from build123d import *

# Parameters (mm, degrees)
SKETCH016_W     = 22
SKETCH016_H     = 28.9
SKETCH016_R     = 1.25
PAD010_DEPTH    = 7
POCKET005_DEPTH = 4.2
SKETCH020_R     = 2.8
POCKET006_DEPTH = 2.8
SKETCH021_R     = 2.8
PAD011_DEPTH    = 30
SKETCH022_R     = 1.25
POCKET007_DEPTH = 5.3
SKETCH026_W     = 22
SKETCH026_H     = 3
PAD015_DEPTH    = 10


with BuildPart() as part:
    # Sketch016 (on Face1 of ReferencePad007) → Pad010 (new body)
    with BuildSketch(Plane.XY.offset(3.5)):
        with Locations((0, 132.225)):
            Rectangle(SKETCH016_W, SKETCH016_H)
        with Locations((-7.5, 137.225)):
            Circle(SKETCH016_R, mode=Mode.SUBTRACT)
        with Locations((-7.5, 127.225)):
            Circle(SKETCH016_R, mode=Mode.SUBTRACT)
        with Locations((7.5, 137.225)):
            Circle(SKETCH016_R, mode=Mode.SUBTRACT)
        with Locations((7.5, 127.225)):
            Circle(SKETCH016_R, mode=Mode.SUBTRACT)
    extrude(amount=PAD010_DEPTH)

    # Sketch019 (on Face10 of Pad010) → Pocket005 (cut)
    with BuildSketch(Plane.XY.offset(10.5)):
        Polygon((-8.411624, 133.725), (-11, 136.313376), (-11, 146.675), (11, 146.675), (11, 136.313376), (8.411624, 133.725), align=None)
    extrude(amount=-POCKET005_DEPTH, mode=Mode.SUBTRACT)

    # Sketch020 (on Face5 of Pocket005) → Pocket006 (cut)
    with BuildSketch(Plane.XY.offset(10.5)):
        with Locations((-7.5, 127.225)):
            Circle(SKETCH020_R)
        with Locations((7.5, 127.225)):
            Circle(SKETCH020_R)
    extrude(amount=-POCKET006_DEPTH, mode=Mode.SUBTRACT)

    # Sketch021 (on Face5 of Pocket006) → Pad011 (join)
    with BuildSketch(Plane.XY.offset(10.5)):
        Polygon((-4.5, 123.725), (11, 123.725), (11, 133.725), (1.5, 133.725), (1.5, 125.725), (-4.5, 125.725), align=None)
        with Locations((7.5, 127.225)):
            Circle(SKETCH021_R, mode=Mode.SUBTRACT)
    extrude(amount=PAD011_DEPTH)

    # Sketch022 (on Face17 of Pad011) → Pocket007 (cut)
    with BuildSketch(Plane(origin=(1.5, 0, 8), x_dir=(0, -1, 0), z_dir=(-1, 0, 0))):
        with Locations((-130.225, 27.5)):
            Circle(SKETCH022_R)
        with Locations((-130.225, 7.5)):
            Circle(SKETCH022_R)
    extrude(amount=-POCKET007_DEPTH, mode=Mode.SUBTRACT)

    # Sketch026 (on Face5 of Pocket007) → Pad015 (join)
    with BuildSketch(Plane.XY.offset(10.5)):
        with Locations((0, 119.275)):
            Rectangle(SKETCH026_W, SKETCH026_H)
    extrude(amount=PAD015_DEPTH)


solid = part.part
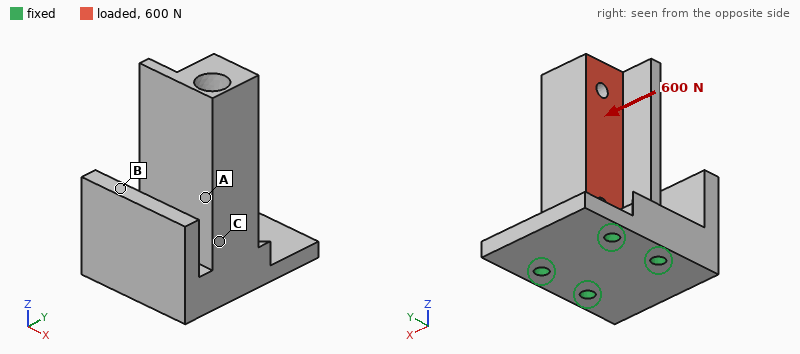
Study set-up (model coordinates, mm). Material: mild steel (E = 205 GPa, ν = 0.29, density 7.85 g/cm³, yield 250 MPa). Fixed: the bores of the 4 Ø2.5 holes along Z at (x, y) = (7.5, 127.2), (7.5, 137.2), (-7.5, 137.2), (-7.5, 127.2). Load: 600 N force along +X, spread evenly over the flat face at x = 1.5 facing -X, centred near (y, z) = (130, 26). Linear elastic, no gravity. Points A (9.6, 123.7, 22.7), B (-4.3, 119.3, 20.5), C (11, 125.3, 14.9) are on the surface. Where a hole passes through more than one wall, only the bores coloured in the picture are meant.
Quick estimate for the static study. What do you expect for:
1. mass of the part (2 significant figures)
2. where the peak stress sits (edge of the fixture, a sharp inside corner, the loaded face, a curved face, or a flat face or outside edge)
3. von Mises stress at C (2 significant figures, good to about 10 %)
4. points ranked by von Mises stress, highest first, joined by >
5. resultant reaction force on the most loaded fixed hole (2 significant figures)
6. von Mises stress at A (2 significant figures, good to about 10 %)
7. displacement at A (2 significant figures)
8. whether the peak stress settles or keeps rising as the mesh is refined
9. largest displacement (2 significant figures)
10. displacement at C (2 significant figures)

48 g
edge of the fixture
48 MPa
C > A > B
720 N
25 MPa
8.6 µm
keeps rising
23 µm
4.5 µm
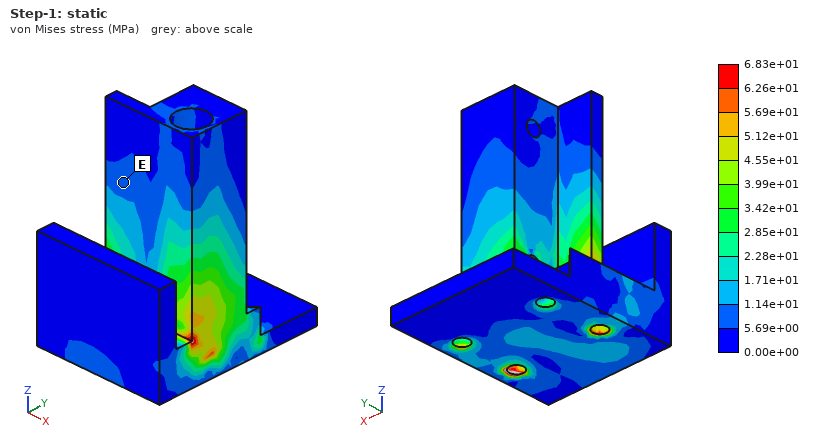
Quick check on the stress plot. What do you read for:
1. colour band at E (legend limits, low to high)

5.69e+00 to 1.14e+01 MPa
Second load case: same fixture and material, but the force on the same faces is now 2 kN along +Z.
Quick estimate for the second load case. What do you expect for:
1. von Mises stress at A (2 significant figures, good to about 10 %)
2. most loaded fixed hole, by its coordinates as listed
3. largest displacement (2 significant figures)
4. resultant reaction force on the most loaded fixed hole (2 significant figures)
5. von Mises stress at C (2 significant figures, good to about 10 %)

24 MPa
(7.5, 127.2)
26 µm
850 N
34 MPa
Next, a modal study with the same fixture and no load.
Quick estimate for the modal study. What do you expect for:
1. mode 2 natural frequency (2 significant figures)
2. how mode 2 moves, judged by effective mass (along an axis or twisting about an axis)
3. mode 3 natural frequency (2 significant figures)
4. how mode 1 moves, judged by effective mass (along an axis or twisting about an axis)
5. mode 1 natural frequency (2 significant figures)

8000 Hz
along X
14 kHz
along Y
5500 Hz
